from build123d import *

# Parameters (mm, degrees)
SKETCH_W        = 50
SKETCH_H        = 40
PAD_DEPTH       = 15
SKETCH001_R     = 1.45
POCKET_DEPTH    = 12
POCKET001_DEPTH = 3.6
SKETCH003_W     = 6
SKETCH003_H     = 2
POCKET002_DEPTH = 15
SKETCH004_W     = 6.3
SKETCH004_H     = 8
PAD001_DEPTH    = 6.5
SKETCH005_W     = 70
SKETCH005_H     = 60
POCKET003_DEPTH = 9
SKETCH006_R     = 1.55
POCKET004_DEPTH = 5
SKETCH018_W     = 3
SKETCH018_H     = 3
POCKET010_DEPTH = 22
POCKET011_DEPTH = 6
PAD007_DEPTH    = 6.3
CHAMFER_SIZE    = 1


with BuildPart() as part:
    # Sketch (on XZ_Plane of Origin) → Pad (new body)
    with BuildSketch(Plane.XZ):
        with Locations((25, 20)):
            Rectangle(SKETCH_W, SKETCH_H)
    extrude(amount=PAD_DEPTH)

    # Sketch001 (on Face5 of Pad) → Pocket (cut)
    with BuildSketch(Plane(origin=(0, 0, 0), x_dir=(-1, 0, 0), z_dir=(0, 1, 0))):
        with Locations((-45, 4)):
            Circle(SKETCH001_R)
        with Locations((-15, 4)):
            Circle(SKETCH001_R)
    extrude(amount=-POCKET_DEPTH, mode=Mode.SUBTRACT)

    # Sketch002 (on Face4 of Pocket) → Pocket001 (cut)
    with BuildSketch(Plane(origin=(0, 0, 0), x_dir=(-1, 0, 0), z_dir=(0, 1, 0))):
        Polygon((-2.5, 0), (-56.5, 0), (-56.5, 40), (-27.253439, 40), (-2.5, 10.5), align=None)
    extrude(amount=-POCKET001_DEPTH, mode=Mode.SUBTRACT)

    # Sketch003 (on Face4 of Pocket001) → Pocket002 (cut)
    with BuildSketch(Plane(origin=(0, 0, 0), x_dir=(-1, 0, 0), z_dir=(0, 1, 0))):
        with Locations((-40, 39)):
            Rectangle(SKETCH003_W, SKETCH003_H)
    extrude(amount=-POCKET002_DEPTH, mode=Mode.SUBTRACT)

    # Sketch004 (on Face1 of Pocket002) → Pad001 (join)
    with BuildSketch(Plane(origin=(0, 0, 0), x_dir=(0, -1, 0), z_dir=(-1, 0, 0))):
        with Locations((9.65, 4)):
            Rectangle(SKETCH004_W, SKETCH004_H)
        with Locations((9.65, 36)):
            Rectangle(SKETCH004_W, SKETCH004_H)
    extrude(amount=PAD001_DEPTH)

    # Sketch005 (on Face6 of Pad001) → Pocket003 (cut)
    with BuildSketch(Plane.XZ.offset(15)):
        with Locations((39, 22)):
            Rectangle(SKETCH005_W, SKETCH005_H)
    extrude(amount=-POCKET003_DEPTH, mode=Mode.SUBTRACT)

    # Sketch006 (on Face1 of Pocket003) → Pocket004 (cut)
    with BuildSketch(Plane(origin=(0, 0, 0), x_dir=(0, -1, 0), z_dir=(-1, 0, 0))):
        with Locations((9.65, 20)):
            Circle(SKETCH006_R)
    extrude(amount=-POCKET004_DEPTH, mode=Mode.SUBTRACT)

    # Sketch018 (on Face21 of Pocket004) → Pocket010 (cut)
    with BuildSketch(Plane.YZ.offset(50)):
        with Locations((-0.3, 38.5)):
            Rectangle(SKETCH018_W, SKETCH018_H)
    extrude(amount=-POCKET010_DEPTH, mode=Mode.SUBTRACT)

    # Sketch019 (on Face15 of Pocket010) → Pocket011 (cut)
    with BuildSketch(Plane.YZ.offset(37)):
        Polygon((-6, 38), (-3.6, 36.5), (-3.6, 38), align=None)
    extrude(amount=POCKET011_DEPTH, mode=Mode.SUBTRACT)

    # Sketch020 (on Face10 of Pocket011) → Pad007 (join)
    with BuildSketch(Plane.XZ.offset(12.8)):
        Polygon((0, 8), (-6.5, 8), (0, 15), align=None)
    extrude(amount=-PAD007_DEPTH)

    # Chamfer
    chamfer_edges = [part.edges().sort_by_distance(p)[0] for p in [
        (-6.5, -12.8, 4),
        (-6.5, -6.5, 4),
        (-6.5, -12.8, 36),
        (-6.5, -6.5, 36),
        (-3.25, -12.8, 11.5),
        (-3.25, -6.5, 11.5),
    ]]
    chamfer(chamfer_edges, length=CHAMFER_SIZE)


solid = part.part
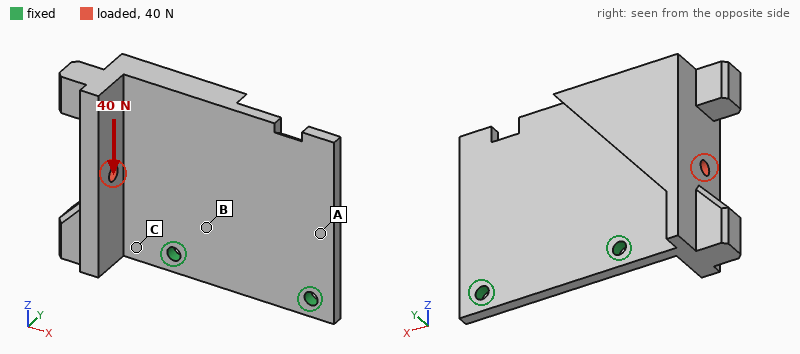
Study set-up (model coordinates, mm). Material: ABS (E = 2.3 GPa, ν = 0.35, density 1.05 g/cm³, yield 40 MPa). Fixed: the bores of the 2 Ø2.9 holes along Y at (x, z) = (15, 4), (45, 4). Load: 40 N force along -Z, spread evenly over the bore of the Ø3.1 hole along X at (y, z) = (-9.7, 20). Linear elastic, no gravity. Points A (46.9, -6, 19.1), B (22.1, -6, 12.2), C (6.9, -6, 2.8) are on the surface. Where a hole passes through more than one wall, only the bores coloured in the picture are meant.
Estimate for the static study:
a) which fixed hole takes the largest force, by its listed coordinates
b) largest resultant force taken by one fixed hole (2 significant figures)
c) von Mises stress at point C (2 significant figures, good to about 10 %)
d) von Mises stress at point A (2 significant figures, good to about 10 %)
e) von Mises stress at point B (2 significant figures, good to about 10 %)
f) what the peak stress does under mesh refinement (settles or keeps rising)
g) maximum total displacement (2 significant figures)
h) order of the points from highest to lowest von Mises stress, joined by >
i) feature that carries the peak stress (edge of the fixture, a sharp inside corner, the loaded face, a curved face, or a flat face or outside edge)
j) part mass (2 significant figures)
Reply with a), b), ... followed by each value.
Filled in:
a) (15, 4)
b) 56 N
c) 7.1 MPa
d) 1.2 MPa
e) 2.8 MPa
f) keeps rising
g) 0.82 mm
h) C > B > A
i) edge of the fixture
j) 9.0 g
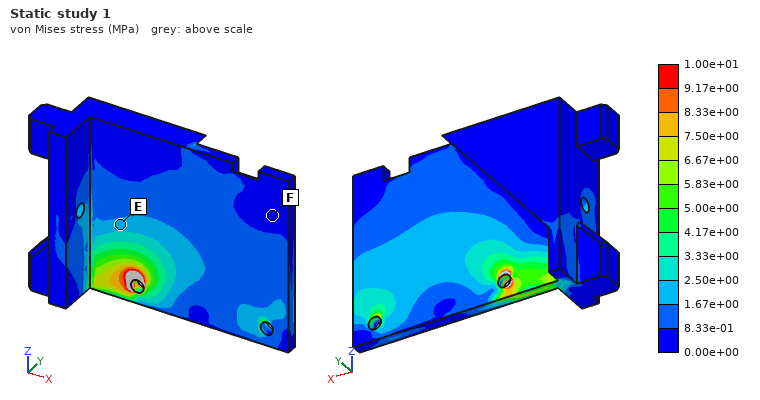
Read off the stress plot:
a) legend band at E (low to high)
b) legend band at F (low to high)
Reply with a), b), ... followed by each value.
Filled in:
a) 1.67e+00 to 2.50e+00 MPa
b) 0.00e+00 to 8.33e-01 MPa
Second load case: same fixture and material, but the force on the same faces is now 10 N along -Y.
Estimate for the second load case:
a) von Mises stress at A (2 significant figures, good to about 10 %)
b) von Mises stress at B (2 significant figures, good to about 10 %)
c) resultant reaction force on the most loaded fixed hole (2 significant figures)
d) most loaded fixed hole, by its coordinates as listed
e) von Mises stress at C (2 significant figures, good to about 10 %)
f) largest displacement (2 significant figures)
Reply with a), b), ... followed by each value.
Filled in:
a) 1.2 MPa
b) 2.8 MPa
c) 12 N
d) (15, 4)
e) 4.8 MPa
f) 0.80 mm
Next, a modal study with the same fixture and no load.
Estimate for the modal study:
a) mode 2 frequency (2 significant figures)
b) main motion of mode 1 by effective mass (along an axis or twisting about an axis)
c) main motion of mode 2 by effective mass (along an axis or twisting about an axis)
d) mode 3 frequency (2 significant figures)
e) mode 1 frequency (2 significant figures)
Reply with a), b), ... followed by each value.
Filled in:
a) 600 Hz
b) along Y
c) twisting about Z
d) 1300 Hz
e) 280 Hz
